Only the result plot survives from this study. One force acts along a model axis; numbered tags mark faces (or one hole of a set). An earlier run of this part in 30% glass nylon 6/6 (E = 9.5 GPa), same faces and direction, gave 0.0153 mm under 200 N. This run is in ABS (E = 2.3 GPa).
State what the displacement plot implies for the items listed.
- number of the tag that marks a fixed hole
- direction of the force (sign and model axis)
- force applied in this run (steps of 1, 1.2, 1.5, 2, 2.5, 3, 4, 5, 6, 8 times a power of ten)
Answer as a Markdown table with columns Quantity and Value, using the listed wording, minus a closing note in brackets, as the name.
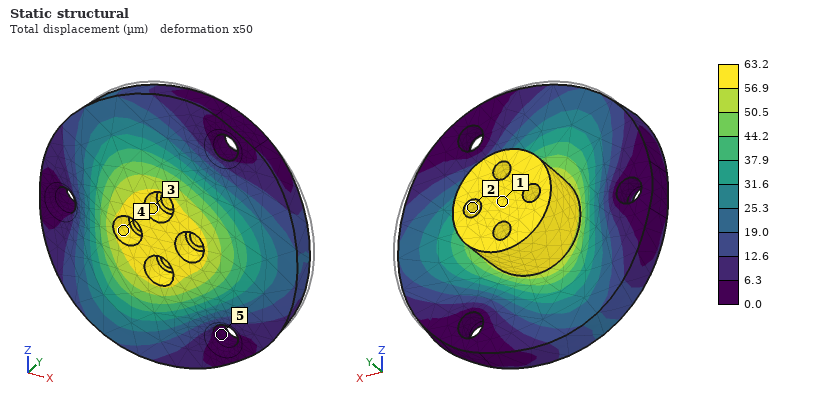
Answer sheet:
| Quantity | Value |
|---|---|
| number of the tag that marks a fixed hole | 5 |
| direction of the force | -Y |
| force applied in this run | 200 N |
